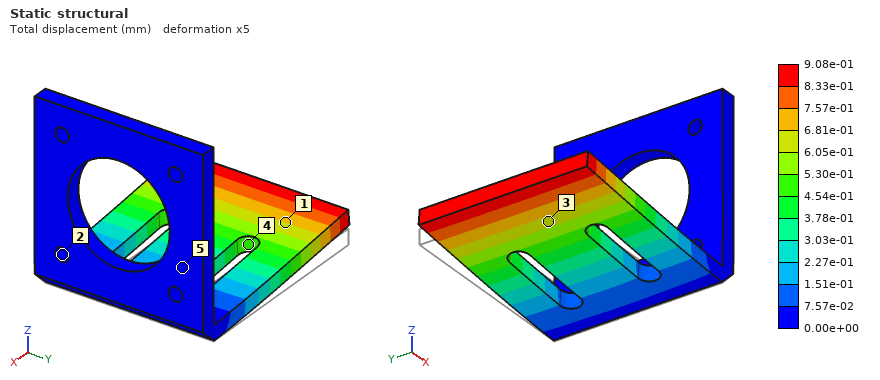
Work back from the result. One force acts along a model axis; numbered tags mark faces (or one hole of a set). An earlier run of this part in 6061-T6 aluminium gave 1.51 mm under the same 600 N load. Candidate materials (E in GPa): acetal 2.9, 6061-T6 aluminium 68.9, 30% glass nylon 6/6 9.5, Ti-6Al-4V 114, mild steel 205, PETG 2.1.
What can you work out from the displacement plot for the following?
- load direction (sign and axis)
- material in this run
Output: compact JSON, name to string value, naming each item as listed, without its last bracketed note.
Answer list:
{"load direction": "+Z", "material in this run": "Ti-6Al-4V"}
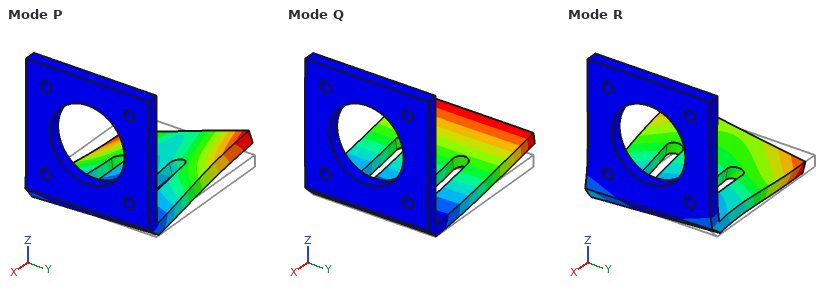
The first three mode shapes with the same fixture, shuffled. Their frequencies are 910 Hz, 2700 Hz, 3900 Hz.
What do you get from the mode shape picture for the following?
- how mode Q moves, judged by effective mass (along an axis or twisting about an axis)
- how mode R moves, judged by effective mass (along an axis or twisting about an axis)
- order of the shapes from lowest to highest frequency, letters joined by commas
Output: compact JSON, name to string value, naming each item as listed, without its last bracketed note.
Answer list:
{"how mode Q moves, judged by effective mass": "along Z", "how mode R moves, judged by effective mass": "along Y", "order of the shapes from lowest to highest frequency, letters joined by commas": "Q, P, R"}
